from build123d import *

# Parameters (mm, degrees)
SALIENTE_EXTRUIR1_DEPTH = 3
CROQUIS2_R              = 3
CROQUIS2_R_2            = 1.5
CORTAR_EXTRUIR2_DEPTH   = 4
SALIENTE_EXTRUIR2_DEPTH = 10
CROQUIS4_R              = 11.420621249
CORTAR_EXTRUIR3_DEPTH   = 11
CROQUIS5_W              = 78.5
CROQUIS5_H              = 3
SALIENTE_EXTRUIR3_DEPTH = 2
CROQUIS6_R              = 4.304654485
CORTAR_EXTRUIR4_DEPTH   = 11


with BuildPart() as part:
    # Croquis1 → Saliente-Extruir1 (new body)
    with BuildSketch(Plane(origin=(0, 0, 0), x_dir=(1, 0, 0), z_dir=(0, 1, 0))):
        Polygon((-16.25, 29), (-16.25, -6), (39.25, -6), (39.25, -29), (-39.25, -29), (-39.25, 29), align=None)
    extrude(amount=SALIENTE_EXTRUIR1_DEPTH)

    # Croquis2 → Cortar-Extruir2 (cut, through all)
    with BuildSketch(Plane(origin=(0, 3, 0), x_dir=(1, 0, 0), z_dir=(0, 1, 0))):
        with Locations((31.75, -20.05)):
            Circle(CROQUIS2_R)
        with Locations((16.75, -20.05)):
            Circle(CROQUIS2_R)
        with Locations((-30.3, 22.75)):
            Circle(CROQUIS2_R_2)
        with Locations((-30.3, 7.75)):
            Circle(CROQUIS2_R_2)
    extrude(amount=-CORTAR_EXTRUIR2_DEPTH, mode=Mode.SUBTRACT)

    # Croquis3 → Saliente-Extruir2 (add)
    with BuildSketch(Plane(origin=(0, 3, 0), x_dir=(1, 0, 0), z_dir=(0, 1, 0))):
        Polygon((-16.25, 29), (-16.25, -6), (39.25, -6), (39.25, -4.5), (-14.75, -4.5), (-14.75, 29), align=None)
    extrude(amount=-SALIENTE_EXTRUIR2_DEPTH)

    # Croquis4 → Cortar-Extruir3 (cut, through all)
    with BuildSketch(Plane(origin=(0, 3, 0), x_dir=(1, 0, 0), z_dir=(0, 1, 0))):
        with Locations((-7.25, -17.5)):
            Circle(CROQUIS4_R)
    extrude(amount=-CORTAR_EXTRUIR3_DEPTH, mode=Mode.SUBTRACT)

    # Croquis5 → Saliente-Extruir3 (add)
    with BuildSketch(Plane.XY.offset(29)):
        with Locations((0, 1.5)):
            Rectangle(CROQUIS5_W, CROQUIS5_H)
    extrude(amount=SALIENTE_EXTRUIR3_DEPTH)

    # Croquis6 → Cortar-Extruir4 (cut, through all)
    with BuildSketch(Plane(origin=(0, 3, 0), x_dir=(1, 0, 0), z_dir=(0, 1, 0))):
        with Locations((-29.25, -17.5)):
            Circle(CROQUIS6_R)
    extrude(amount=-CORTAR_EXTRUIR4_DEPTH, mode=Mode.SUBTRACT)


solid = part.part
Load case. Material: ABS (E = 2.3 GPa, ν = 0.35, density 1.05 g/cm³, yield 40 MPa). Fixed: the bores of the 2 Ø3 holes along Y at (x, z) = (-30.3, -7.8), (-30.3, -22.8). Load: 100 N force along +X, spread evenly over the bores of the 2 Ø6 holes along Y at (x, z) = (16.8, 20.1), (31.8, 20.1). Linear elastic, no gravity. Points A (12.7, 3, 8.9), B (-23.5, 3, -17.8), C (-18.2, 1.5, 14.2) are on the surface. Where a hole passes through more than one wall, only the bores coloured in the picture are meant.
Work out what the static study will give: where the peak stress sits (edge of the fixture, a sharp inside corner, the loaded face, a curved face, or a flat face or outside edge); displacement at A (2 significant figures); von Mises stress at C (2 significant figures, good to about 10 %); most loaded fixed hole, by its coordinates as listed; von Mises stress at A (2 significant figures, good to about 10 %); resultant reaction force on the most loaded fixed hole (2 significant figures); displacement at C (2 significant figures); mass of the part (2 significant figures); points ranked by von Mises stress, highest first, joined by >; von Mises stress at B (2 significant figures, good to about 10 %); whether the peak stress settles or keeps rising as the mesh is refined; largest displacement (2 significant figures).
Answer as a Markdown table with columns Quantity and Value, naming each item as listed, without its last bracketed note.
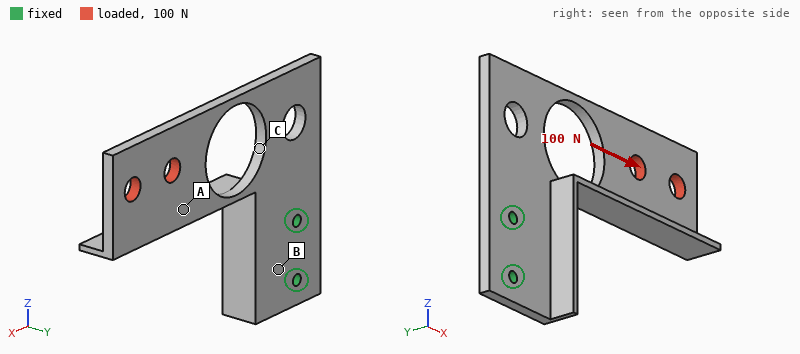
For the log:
| Quantity | Value |
|---|---|
| where the peak stress sits | edge of the fixture |
| displacement at A | 0.59 mm |
| von Mises stress at C | 9.9 MPa |
| most loaded fixed hole, by its coordinates as listed | (-30.3, -7.8) |
| von Mises stress at A | 1.7 MPa |
| resultant reaction force on the most loaded fixed hole | 250 N |
| displacement at C | 0.24 mm |
| mass of the part | 8.4 g |
| points ranked by von Mises stress, highest first, joined by > | C > B > A |
| von Mises stress at B | 4.8 MPa |
| whether the peak stress settles or keeps rising as the mesh is refined | keeps rising |
| largest displacement | 1.1 mm |
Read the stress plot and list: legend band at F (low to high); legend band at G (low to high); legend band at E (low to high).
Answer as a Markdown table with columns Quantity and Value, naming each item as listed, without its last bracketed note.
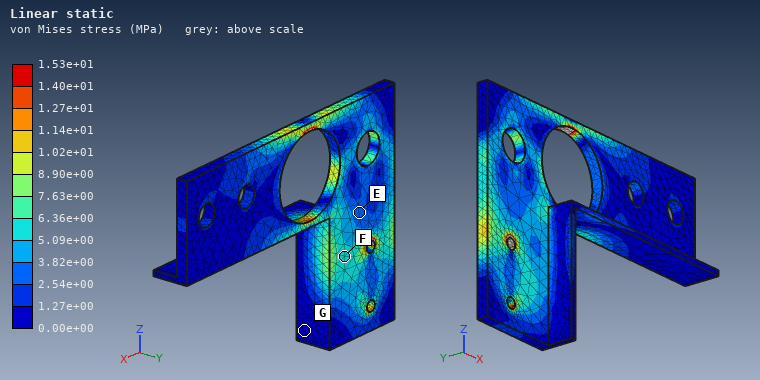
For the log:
| Quantity | Value |
|---|---|
| legend band at F | 5.09e+00 to 6.36e+00 MPa |
| legend band at G | 0.00e+00 to 1.27e+00 MPa |
| legend band at E | 2.54e+00 to 3.82e+00 MPa |
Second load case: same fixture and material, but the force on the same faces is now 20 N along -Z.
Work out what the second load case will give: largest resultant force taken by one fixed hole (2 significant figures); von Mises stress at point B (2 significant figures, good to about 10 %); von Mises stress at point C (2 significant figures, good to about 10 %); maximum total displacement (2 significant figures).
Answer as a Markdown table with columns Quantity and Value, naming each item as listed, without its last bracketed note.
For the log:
| Quantity | Value |
|---|---|
| largest resultant force taken by one fixed hole | 63 N |
| von Mises stress at point B | 2.0 MPa |
| von Mises stress at point C | 5.3 MPa |
| maximum total displacement | 0.91 mm |
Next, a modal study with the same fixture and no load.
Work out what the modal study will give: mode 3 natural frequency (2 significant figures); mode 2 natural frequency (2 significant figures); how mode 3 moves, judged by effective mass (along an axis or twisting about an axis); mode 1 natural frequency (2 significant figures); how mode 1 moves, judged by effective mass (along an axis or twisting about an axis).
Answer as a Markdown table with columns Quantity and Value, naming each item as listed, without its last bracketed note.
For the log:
| Quantity | Value |
|---|---|
| mode 3 natural frequency | 490 Hz |
| mode 2 natural frequency | 390 Hz |
| how mode 3 moves, judged by effective mass | along Z |
| mode 1 natural frequency | 130 Hz |
| how mode 1 moves, judged by effective mass | along Y |
